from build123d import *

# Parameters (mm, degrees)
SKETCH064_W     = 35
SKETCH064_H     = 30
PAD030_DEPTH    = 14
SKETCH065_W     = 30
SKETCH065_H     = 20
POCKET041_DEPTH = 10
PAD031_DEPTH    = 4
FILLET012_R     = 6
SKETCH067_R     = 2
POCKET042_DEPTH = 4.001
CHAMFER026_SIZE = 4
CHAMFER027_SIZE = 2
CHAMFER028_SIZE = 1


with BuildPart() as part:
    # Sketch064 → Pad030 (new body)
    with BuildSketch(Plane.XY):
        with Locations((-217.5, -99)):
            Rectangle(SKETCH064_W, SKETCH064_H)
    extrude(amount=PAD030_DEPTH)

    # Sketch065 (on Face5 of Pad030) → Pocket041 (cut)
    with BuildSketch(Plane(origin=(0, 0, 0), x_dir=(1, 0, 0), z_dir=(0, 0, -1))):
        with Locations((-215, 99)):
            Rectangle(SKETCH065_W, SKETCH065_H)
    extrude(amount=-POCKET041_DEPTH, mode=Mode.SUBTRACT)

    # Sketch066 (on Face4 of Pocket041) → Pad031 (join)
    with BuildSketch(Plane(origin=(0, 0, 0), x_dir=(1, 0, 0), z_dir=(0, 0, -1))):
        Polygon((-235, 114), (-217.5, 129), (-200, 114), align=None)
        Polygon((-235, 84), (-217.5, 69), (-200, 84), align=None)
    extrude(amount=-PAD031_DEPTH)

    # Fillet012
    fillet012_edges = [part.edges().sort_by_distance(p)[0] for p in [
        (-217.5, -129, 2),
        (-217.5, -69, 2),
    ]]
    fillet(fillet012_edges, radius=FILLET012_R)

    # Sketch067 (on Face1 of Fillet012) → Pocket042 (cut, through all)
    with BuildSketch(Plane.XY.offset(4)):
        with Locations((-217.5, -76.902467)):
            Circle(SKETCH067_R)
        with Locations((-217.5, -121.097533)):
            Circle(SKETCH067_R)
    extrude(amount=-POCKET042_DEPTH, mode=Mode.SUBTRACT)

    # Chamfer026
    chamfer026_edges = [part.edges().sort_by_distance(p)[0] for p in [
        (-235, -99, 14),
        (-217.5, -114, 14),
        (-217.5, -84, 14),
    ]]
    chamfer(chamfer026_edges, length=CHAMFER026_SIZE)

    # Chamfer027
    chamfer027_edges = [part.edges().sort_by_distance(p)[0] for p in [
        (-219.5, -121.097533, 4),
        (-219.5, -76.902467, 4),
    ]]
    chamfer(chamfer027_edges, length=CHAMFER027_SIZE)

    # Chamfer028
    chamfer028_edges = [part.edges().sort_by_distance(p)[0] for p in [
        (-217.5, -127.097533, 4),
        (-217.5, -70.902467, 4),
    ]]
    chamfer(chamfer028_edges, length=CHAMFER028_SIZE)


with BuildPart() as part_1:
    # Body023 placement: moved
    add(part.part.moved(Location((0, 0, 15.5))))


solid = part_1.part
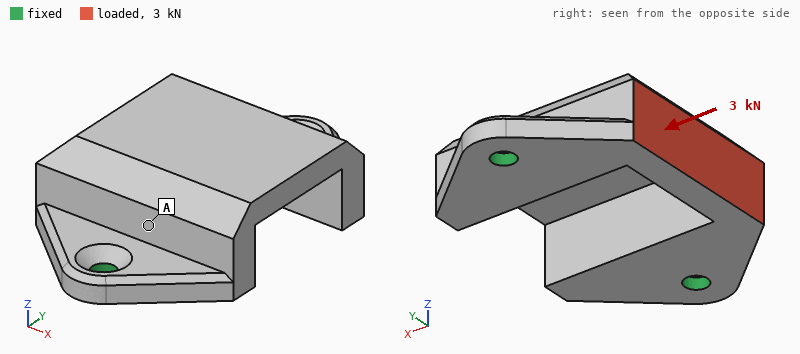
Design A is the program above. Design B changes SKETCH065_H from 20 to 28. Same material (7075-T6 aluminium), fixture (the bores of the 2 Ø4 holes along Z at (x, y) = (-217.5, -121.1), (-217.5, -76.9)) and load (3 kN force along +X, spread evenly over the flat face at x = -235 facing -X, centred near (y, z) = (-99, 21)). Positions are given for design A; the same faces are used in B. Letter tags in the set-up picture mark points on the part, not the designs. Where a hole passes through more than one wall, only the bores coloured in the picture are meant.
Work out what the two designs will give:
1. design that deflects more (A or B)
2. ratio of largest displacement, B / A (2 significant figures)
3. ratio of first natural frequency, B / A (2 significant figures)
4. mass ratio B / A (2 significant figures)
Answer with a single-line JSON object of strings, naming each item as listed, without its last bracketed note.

{"design that deflects more": "B", "ratio of largest displacement, B / A": "1.1", "ratio of first natural frequency, B / A": "1.0", "mass ratio B / A": "0.75"}
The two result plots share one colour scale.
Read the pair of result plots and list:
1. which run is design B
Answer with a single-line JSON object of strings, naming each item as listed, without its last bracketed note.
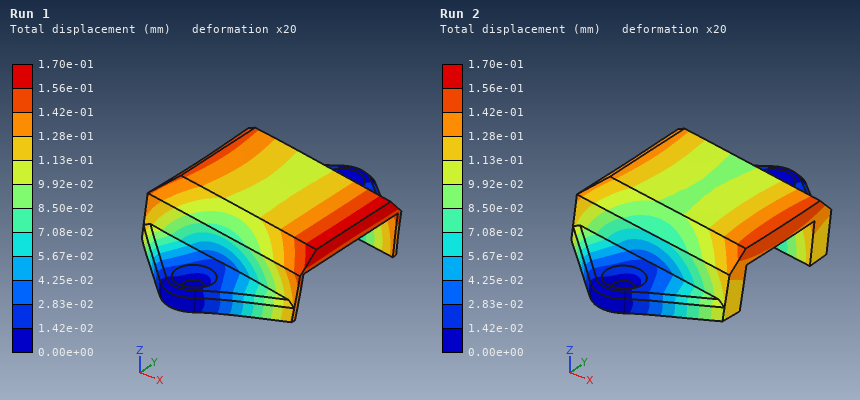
{"which run is design B": "Run 1"}
